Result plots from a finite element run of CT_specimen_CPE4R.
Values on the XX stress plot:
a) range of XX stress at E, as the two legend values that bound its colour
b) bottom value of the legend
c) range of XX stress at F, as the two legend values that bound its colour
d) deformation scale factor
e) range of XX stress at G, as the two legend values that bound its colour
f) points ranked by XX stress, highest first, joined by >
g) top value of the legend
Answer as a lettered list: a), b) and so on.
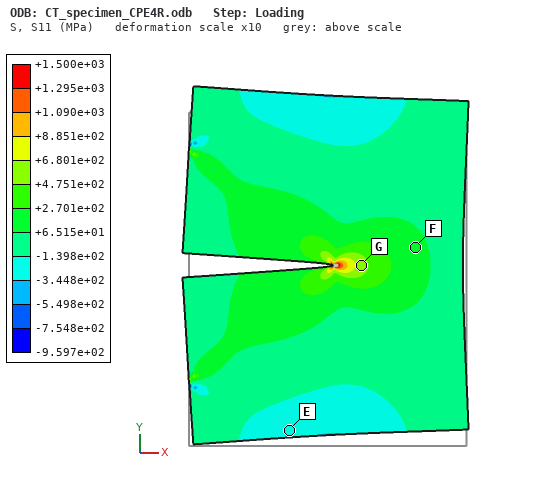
a) -3.448e+02 to -1.398e+02 MPa
b) -9.597e+02 MPa
c) +6.515e+01 to +2.701e+02 MPa
d) 10
e) +4.751e+02 to +6.801e+02 MPa
f) G > F > E
g) +1.500e+03 MPa
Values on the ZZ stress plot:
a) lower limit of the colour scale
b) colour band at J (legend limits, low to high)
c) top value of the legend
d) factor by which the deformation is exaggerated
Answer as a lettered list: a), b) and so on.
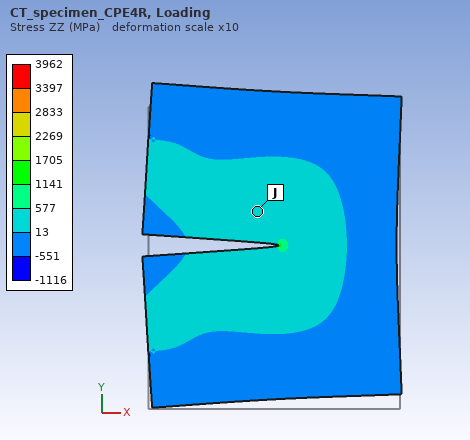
a) -1116 MPa
b) 13 to 577 MPa
c) 3962 MPa
d) 10
